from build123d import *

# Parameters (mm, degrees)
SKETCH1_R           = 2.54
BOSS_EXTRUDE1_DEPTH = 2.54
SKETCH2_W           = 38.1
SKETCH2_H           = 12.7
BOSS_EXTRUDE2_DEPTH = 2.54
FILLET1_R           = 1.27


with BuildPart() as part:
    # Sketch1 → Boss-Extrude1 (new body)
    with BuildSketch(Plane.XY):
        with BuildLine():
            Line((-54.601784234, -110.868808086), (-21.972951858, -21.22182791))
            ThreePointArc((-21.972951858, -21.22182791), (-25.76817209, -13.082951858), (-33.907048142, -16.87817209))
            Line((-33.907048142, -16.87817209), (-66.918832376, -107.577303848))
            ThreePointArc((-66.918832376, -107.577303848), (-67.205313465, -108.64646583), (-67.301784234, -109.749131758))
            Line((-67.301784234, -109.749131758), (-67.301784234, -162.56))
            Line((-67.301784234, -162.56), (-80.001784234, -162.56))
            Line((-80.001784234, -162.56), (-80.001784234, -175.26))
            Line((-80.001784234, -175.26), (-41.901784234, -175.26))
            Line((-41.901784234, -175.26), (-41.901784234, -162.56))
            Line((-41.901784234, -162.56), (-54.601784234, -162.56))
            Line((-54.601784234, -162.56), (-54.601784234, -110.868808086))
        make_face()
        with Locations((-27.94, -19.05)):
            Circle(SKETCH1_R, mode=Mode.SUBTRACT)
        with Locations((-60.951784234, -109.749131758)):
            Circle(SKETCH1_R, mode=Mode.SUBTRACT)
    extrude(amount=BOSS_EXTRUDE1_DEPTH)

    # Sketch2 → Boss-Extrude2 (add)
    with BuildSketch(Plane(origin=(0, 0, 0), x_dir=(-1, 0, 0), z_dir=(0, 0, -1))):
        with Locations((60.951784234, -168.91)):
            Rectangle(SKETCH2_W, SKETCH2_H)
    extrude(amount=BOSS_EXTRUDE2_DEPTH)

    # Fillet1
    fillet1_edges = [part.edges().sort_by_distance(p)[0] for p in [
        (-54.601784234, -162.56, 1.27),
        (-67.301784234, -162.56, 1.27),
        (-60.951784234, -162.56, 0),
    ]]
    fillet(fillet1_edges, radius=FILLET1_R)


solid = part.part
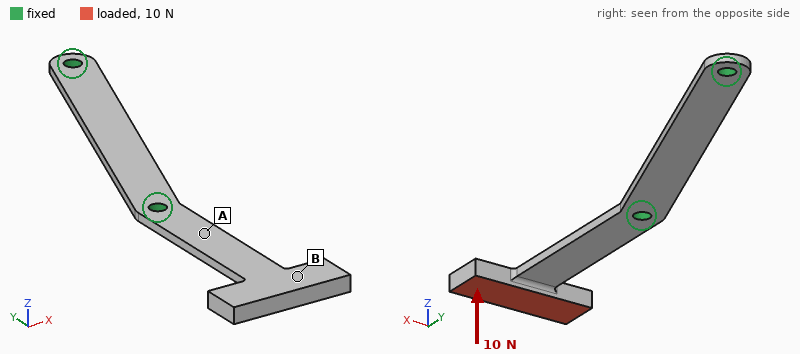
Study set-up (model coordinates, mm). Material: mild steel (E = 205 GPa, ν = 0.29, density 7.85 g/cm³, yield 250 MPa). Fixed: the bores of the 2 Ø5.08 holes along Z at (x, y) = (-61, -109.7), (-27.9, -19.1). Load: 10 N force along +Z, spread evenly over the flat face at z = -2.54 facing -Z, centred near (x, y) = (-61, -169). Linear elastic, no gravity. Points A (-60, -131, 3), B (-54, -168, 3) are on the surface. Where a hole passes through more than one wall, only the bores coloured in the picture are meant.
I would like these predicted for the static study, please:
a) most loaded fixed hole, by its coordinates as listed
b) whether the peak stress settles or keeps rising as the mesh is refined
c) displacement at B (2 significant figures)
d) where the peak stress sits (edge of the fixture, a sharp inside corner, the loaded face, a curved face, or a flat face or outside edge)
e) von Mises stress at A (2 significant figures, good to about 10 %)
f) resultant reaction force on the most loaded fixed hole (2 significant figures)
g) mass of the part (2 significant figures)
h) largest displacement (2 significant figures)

(-61, -109.7)
keeps rising
0.17 mm
edge of the fixture
27 MPa
10.0 N
58 g
0.21 mm
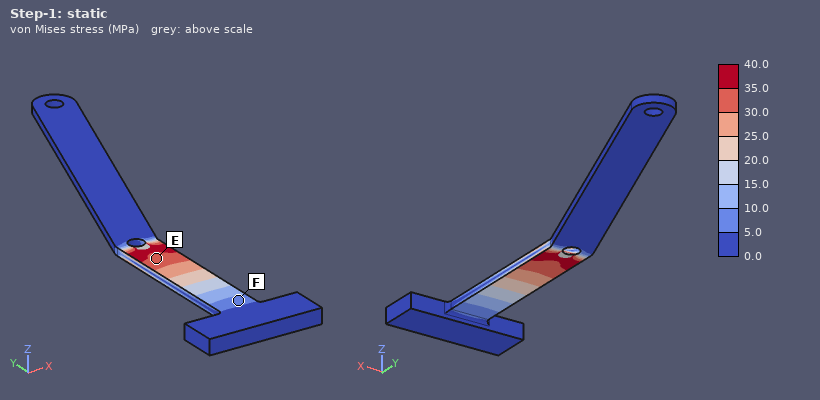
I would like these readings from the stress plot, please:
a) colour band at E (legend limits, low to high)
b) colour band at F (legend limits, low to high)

30.0 to 35.0 MPa
5.0 to 10.0 MPa
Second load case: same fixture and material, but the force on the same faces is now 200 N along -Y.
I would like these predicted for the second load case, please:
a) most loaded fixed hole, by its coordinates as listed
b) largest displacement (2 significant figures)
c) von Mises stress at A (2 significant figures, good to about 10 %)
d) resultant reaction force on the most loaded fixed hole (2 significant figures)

(-61, -109.7)
0.42 mm
49 MPa
200 N
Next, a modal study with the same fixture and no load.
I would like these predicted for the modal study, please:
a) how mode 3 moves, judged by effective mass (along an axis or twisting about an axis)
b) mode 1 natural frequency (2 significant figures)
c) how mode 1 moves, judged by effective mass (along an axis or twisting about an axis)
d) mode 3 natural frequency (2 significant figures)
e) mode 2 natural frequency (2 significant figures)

along X
260 Hz
along Z
1100 Hz
990 Hz
